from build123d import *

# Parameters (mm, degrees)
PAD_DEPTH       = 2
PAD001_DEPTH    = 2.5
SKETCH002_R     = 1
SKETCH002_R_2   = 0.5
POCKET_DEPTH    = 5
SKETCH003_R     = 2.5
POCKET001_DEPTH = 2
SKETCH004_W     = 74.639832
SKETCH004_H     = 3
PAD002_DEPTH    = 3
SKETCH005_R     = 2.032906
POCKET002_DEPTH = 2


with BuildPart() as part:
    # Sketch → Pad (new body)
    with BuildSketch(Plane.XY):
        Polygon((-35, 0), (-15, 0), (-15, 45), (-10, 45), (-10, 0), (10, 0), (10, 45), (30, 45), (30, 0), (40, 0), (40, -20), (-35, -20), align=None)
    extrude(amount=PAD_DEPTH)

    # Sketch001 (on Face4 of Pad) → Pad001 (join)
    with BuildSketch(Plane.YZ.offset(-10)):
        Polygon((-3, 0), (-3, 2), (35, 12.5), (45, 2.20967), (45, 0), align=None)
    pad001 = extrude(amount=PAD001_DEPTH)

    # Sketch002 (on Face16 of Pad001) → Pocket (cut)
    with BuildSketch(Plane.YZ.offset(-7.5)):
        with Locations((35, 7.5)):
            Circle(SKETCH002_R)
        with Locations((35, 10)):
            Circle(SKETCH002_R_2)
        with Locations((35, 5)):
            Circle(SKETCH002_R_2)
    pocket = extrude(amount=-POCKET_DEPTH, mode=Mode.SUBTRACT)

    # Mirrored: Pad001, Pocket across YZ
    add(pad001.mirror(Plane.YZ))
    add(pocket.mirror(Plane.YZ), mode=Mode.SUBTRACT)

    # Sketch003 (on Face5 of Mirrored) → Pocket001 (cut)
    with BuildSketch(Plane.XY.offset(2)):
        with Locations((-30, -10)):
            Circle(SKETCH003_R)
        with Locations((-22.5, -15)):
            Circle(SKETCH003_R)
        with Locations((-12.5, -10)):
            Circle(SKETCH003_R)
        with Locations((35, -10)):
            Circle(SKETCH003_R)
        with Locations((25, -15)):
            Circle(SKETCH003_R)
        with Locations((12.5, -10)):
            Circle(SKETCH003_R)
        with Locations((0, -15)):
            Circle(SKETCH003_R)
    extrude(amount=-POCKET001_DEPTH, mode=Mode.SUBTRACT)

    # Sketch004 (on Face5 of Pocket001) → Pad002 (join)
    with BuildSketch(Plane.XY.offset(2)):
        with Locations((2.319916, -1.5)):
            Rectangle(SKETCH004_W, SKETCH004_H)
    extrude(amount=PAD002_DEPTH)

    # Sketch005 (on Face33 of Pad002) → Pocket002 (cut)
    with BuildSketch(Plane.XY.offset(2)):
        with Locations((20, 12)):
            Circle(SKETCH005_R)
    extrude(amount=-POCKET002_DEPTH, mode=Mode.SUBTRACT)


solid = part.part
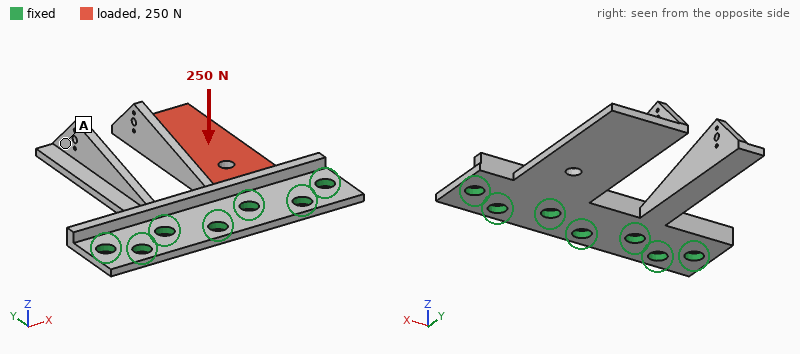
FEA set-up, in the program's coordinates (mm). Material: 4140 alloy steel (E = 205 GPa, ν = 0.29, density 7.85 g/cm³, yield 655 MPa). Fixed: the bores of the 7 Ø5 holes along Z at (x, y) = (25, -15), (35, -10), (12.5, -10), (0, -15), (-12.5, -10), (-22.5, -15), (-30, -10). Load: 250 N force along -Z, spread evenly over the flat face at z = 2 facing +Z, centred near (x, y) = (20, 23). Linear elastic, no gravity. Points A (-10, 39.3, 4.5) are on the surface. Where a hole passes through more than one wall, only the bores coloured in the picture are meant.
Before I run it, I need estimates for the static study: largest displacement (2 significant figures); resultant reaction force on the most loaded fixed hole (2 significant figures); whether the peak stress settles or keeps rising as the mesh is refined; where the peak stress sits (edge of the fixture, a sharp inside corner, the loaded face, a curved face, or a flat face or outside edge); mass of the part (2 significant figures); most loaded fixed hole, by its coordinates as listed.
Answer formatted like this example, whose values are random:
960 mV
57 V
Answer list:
0.89 mm
300 N
keeps rising
edge of the fixture
57 g
(12.5, -10)
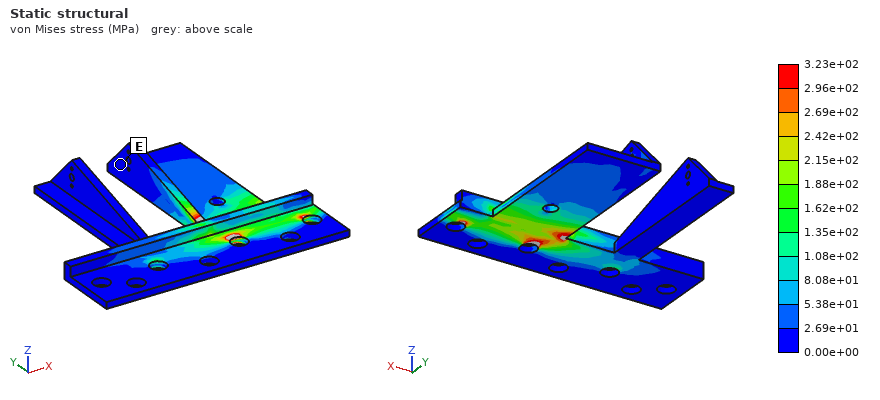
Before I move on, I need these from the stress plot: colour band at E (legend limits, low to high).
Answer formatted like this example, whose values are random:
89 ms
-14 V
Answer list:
0.00e+00 to 2.69e+01 MPa
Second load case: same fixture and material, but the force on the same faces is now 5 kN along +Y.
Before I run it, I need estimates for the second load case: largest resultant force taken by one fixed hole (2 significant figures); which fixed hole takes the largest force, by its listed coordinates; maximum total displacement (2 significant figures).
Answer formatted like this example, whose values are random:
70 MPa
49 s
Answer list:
2.1 kN
(12.5, -10)
0.72 mm
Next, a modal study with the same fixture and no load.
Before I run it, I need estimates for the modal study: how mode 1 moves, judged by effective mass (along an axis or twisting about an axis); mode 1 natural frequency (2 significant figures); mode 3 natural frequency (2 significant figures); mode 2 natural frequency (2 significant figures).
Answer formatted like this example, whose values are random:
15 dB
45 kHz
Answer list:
along Z
710 Hz
2100 Hz
840 Hz
